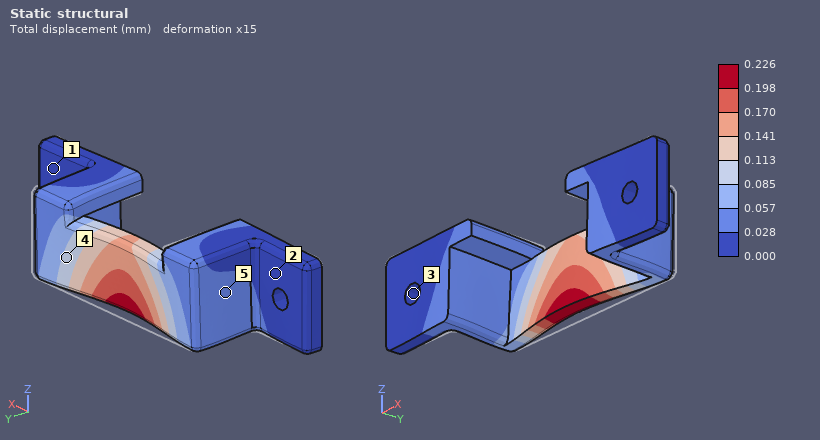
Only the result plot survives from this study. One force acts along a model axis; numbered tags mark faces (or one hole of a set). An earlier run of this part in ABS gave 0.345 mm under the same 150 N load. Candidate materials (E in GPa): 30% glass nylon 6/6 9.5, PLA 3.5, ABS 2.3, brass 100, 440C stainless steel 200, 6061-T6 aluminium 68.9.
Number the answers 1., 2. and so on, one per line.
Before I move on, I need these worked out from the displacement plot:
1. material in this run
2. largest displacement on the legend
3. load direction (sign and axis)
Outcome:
1. PLA
2. 0.226 mm
3. -Y
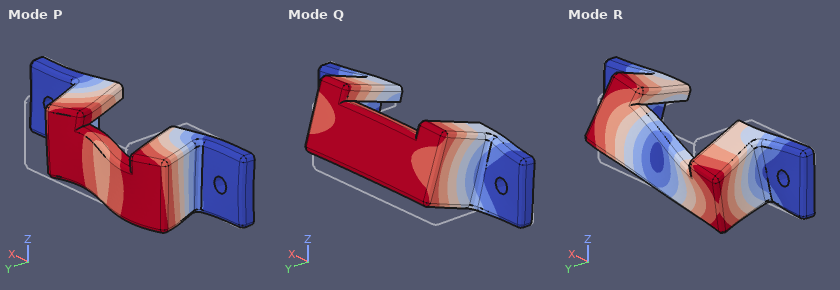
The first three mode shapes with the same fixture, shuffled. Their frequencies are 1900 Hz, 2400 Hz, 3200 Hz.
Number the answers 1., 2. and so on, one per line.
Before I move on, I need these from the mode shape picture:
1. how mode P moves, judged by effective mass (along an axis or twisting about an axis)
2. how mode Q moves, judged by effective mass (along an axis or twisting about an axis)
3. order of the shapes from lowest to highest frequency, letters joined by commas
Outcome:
1. along X
2. along Z
3. Q, P, R
